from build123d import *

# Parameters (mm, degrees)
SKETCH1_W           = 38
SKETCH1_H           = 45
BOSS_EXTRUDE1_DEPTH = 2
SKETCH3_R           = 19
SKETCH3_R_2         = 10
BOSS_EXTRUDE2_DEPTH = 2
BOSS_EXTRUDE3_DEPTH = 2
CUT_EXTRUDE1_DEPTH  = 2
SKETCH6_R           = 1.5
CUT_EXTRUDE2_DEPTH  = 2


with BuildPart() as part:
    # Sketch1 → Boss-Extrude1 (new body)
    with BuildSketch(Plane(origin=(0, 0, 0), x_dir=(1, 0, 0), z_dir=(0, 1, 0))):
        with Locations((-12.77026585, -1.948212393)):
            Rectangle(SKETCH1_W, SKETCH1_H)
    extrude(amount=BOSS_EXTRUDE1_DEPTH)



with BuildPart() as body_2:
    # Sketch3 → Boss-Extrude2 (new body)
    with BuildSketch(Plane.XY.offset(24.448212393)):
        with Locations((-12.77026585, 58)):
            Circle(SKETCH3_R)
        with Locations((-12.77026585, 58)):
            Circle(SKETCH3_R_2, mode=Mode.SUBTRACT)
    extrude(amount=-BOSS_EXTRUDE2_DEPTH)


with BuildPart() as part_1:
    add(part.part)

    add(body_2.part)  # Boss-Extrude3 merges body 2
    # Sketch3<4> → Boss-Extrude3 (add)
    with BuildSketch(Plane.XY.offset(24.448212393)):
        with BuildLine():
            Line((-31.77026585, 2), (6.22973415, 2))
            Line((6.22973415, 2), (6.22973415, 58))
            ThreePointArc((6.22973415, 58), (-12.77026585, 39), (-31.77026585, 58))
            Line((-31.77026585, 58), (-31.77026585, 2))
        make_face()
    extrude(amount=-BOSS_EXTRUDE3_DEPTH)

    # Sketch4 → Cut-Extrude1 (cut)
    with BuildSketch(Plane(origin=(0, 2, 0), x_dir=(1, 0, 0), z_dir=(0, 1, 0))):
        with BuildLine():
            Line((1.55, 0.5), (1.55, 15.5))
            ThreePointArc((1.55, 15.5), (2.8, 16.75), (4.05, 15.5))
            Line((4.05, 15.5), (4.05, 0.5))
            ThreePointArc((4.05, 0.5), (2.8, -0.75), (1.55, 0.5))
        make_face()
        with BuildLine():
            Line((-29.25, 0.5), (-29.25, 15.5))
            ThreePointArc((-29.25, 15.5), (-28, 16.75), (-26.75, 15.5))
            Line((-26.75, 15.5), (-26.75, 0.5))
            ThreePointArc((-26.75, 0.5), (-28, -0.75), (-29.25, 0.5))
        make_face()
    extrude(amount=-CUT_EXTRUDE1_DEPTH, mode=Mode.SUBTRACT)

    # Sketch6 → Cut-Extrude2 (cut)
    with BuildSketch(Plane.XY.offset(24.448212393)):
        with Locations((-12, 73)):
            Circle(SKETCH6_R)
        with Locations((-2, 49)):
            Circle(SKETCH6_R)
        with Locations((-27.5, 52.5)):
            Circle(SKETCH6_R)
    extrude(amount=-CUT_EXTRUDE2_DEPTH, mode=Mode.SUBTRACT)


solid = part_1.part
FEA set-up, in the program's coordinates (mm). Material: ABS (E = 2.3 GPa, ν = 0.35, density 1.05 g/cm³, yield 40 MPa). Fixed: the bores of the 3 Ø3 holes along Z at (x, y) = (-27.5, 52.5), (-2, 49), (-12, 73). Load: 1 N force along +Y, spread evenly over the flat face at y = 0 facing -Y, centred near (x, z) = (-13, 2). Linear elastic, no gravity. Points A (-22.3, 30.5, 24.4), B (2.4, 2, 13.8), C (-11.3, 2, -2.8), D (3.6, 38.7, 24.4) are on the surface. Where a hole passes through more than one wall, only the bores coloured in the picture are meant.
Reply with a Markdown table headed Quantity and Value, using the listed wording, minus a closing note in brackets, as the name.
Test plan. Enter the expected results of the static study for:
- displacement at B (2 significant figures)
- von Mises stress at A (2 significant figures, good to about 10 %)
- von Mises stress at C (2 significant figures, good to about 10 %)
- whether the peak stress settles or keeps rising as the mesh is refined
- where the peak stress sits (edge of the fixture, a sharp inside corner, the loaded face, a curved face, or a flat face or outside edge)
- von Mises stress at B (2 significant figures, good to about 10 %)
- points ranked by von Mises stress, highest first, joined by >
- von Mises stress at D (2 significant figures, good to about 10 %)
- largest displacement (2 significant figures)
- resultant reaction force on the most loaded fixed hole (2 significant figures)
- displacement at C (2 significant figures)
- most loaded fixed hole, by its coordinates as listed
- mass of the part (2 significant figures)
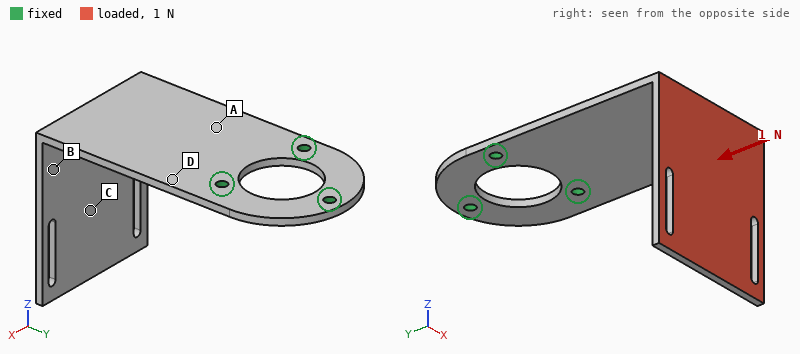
| Quantity | Value |
|---|---|
| displacement at B | 0.46 mm |
| von Mises stress at A | 0.76 MPa |
| von Mises stress at C | 0.14 MPa |
| whether the peak stress settles or keeps rising as the mesh is refined | keeps rising |
| where the peak stress sits | edge of the fixture |
| von Mises stress at B | 0.45 MPa |
| points ranked by von Mises stress, highest first, joined by > | D > A > B > C |
| von Mises stress at D | 0.96 MPa |
| largest displacement | 1.0 mm |
| resultant reaction force on the most loaded fixed hole | 0.56 N |
| displacement at C | 0.68 mm |
| most loaded fixed hole, by its coordinates as listed | (-2, 49) |
| mass of the part | 8.4 g |
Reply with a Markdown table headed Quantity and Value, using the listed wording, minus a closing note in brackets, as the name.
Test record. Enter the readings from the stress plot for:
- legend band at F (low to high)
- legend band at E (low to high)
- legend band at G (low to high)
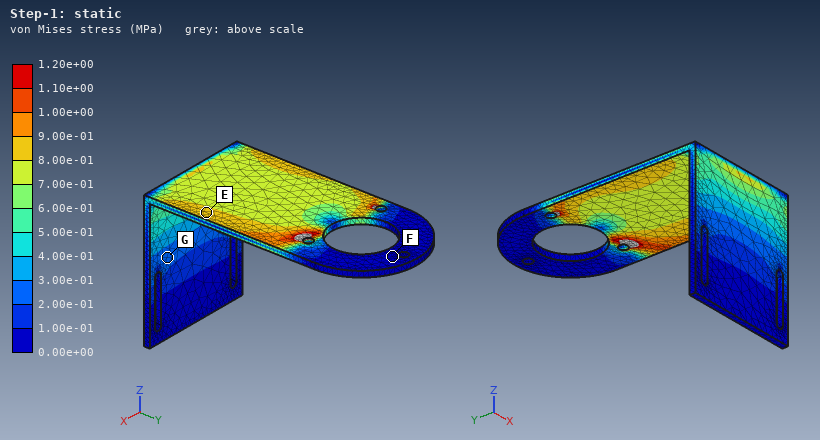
| Quantity | Value |
|---|---|
| legend band at F | 0.00e+00 to 1.00e-01 MPa |
| legend band at E | 8.00e-01 to 9.00e-01 MPa |
| legend band at G | 2.00e-01 to 3.00e-01 MPa |
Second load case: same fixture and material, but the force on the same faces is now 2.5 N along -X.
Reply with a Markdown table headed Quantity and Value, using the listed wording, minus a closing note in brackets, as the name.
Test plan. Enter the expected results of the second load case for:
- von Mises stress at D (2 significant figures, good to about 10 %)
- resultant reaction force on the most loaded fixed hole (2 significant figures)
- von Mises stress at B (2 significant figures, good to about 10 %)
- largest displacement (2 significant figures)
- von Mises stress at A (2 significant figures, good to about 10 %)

| Quantity | Value |
|---|---|
| von Mises stress at D | 1.4 MPa |
| resultant reaction force on the most loaded fixed hole | 4.9 N |
| von Mises stress at B | 0.56 MPa |
| largest displacement | 1.1 mm |
| von Mises stress at A | 1.5 MPa |
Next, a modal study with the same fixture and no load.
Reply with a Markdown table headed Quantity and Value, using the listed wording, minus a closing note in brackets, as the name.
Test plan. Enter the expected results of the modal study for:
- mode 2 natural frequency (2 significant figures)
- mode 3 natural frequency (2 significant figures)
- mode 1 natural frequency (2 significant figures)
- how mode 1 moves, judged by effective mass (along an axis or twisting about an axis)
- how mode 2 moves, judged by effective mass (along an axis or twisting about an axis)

| Quantity | Value |
|---|---|
| mode 2 natural frequency | 150 Hz |
| mode 3 natural frequency | 220 Hz |
| mode 1 natural frequency | 73 Hz |
| how mode 1 moves, judged by effective mass | along Z |
| how mode 2 moves, judged by effective mass | along X |
